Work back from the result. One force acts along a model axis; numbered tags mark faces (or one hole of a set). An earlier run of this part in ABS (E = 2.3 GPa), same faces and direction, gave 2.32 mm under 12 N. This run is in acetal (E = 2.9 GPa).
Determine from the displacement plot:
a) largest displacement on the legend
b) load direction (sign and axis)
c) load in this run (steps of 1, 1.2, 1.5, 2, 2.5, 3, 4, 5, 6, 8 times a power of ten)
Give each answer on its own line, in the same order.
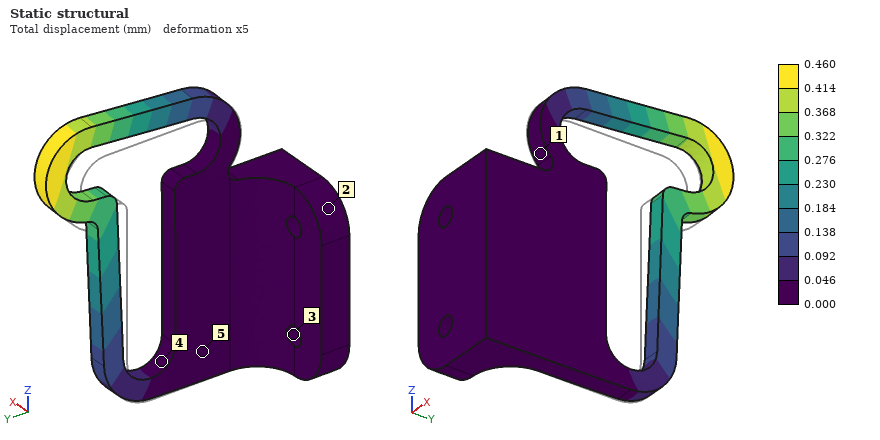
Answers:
0.460 mm
+X
3 N
